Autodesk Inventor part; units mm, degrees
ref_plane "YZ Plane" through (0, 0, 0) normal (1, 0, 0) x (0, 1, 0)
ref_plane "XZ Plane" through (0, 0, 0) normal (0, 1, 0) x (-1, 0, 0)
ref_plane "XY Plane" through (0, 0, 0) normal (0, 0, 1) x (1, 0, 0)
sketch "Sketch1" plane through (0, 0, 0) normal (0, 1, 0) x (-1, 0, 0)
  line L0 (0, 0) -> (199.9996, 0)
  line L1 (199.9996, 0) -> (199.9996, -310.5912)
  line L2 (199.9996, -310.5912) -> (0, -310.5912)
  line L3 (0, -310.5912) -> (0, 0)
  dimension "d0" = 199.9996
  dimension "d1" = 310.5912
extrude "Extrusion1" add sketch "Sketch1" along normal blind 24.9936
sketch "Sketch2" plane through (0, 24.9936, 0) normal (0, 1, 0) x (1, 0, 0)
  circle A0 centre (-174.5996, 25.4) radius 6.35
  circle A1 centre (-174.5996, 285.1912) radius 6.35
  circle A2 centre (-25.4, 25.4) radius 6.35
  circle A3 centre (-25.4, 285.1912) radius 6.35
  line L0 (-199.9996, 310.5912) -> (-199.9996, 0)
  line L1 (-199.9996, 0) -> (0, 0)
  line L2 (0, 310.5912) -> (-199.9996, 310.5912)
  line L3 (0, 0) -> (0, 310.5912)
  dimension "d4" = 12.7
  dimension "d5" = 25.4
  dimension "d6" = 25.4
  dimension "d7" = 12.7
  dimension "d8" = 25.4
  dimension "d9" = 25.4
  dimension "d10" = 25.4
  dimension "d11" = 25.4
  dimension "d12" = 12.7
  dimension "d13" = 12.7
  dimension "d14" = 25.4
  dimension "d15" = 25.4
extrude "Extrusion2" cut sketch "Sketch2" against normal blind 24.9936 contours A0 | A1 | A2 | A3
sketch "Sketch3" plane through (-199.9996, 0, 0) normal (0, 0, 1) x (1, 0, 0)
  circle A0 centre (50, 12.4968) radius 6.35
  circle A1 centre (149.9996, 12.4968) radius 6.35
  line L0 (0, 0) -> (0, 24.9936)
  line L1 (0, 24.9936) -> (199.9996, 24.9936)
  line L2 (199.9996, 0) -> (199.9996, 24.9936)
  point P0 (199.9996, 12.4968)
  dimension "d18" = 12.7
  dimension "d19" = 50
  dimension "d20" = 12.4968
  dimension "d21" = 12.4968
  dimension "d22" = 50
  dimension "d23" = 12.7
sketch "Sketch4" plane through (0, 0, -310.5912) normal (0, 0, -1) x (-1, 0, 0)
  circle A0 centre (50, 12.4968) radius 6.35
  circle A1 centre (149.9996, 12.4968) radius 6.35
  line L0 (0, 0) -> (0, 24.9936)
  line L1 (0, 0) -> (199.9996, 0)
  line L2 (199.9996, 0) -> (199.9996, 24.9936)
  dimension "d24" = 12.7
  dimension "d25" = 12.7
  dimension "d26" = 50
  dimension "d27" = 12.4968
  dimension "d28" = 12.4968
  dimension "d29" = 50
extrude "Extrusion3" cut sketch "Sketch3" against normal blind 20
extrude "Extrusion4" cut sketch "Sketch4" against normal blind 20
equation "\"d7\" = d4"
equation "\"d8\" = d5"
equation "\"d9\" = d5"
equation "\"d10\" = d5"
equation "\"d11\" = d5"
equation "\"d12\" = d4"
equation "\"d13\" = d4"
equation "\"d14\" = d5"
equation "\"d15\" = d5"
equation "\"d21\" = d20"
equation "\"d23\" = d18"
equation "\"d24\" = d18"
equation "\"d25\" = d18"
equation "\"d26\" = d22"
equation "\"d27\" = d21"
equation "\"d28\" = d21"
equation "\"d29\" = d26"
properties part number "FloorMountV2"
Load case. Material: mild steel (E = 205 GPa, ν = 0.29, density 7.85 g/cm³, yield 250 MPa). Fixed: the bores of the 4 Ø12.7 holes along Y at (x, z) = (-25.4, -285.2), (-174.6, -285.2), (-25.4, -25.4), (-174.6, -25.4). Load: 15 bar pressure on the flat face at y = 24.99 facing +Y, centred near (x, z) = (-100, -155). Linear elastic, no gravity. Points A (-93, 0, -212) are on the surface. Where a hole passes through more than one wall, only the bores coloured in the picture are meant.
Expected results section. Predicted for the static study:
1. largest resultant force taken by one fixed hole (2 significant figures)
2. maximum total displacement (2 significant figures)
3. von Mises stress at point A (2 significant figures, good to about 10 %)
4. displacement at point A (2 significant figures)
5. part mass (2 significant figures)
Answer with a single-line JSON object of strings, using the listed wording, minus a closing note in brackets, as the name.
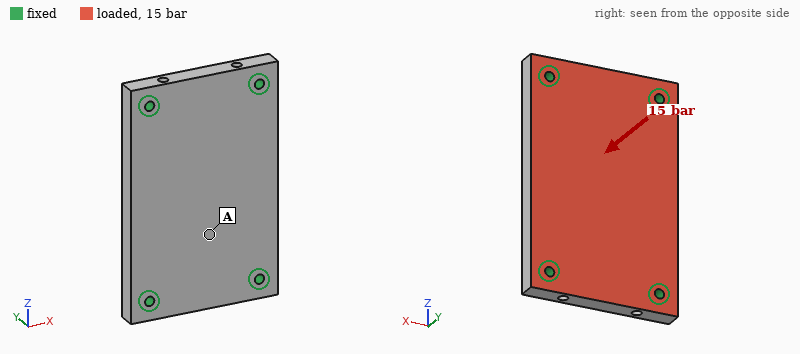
{"largest resultant force taken by one fixed hole": "23 kN", "maximum total displacement": "0.11 mm", "von Mises stress at point A": "25 MPa", "displacement at point A": "0.081 mm", "part mass": "12 kg"}
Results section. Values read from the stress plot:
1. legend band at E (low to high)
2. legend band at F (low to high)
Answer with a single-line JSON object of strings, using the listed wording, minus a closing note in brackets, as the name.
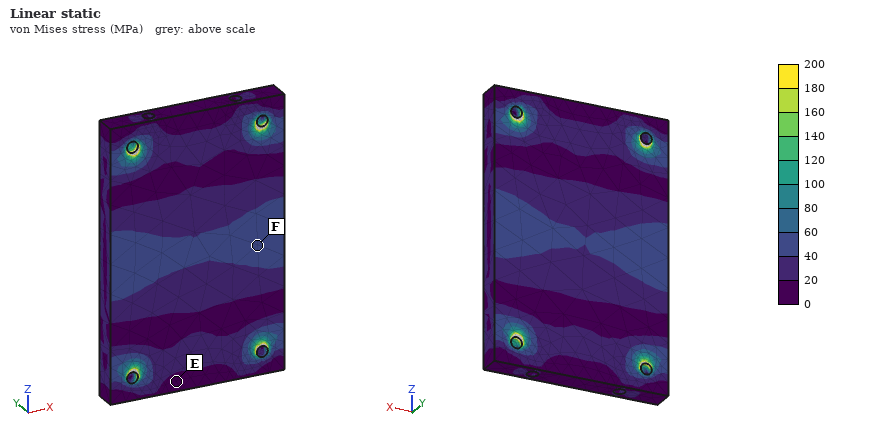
{"legend band at E": "0 to 20 MPa", "legend band at F": "40 to 60 MPa"}
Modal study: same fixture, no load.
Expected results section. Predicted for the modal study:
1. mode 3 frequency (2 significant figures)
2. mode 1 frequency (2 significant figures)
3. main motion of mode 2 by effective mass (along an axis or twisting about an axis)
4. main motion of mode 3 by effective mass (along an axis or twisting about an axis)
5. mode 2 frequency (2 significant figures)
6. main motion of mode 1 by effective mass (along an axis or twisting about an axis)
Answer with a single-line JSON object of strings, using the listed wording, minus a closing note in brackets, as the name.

{"mode 3 frequency": "3800 Hz", "mode 1 frequency": "1500 Hz", "main motion of mode 2 by effective mass": "twisting about Z", "main motion of mode 3 by effective mass": "twisting about X", "mode 2 frequency": "2300 Hz", "main motion of mode 1 by effective mass": "along Y"}
